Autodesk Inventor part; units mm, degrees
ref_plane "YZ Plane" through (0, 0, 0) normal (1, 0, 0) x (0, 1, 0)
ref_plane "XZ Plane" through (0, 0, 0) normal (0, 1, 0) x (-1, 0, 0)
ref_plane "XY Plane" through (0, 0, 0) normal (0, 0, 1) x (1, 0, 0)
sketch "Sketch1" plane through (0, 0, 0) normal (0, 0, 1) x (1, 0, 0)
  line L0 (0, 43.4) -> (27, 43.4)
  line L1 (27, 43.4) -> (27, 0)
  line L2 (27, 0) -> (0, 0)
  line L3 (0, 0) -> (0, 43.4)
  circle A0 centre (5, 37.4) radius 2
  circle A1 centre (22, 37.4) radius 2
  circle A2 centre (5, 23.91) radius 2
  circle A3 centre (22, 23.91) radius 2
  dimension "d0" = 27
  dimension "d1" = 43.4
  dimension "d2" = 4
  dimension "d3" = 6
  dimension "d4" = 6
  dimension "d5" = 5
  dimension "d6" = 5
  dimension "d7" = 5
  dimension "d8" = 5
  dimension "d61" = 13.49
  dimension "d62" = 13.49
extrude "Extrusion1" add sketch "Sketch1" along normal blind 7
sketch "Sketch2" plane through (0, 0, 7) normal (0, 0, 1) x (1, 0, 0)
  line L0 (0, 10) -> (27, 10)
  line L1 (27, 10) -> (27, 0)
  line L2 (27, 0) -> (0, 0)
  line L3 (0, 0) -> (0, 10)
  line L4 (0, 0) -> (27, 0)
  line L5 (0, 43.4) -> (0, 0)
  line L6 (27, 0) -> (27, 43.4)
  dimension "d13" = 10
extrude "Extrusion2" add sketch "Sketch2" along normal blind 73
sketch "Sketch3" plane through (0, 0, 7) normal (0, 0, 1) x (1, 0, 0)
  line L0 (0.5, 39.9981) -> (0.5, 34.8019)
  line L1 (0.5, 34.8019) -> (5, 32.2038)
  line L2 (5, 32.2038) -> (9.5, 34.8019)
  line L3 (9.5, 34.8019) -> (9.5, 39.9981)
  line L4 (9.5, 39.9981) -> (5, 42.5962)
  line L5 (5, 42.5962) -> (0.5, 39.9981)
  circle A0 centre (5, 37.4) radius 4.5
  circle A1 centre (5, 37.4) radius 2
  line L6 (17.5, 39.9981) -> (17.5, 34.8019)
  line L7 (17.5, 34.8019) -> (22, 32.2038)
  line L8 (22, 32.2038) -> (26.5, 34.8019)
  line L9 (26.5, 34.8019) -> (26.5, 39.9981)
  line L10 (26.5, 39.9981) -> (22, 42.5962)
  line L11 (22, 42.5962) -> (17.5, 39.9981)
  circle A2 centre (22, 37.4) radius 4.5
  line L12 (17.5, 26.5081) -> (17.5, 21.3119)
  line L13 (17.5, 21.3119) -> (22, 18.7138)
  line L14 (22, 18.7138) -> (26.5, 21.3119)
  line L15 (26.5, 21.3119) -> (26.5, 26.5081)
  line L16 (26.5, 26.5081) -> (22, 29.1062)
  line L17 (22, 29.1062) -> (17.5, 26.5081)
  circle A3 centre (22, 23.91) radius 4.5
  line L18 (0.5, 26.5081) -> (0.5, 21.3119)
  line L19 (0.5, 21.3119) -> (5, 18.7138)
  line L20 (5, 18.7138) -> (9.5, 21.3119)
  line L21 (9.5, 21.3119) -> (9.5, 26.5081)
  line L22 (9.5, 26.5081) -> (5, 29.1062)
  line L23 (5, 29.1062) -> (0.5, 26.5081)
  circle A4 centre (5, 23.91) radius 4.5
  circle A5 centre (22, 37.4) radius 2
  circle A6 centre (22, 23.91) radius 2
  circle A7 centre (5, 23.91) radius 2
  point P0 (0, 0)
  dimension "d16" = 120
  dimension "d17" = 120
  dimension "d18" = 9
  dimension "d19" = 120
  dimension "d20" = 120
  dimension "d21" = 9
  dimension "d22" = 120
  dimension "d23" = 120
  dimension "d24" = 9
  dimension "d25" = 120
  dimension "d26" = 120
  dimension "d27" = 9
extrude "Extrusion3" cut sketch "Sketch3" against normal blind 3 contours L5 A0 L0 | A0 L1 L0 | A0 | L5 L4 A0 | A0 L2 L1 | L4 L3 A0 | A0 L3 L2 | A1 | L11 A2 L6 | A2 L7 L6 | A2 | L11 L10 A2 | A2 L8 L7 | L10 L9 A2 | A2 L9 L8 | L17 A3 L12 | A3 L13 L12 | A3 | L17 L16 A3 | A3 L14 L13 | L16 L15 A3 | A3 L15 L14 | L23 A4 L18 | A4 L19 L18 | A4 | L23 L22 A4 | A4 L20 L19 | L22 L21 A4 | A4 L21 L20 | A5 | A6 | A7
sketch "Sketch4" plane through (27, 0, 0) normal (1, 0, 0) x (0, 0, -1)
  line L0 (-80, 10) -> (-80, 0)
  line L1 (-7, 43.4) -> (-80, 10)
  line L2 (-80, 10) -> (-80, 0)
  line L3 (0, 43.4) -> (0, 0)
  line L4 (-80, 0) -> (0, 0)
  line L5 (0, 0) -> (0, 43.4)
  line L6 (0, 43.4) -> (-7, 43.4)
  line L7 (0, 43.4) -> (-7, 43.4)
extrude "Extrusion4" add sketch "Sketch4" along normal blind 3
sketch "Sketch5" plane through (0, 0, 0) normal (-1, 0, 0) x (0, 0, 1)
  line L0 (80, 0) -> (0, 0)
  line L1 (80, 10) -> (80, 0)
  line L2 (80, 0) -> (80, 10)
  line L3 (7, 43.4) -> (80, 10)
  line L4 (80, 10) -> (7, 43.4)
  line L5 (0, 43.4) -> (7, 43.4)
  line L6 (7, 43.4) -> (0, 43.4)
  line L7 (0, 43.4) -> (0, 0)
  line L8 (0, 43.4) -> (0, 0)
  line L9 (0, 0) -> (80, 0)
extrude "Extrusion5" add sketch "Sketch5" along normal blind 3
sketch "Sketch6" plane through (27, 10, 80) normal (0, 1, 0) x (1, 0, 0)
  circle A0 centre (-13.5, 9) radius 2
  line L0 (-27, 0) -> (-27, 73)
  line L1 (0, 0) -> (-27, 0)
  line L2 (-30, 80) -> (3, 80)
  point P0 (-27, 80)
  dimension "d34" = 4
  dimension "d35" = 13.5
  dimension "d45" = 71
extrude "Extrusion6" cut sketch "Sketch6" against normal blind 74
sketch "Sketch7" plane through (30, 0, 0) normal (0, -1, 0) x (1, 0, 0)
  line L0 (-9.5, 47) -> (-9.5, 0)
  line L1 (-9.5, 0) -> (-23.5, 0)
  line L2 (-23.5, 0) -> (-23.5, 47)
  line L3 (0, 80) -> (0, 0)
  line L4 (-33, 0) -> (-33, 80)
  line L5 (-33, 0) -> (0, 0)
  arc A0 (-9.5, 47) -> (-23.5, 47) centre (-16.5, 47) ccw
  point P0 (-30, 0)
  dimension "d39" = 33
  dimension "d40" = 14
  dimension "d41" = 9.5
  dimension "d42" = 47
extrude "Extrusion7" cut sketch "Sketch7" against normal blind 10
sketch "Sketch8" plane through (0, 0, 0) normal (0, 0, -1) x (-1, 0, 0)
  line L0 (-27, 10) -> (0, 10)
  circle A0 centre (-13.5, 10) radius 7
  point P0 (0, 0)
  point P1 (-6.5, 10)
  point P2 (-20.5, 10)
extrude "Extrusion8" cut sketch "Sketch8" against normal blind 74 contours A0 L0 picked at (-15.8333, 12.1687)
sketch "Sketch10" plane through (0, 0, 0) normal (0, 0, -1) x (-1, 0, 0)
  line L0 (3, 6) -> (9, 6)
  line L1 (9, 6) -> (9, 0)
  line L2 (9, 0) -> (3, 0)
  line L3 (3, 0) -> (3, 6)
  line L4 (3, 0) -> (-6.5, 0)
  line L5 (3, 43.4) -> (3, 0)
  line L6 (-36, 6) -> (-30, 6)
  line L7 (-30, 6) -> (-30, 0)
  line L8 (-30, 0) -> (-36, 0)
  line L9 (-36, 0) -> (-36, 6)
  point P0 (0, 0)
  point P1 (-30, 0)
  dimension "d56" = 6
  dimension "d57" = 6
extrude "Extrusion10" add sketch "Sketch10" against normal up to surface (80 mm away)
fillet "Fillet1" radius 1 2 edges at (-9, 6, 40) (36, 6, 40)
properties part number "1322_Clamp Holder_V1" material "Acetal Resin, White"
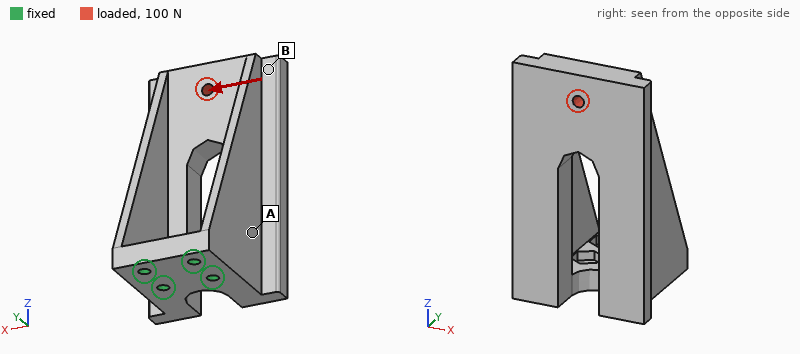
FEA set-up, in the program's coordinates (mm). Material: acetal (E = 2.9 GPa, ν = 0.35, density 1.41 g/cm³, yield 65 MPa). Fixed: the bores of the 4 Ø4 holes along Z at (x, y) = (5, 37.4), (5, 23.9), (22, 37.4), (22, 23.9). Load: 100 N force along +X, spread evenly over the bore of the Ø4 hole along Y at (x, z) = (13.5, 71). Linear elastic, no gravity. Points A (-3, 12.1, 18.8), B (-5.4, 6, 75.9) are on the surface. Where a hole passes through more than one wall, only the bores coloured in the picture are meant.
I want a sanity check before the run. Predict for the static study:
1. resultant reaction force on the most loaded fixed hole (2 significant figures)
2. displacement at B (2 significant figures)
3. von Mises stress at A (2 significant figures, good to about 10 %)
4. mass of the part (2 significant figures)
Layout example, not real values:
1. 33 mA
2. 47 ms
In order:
1. 270 N
2. 1.0 mm
3. 3.3 MPa
4. 54 g
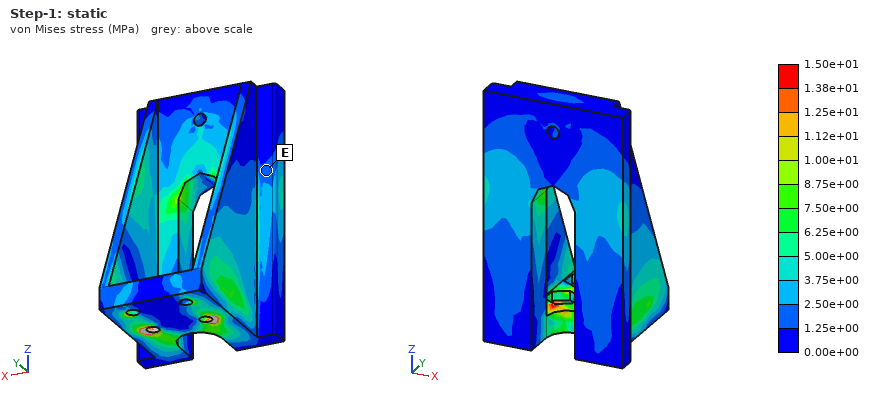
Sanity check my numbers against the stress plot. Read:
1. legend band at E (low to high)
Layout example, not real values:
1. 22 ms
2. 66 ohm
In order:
1. 1.25e+00 to 2.50e+00 MPa
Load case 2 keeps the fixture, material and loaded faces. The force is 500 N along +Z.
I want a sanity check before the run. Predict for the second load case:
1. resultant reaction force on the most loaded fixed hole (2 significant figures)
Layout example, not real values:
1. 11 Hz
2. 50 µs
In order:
1. 500 N
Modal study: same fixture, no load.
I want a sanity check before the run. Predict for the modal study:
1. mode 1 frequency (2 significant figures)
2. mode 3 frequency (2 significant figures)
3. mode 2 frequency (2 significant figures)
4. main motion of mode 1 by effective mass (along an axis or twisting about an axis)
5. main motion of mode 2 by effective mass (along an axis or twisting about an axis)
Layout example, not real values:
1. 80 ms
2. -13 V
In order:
1. 350 Hz
2. 1000 Hz
3. 450 Hz
4. along X
5. along Y
